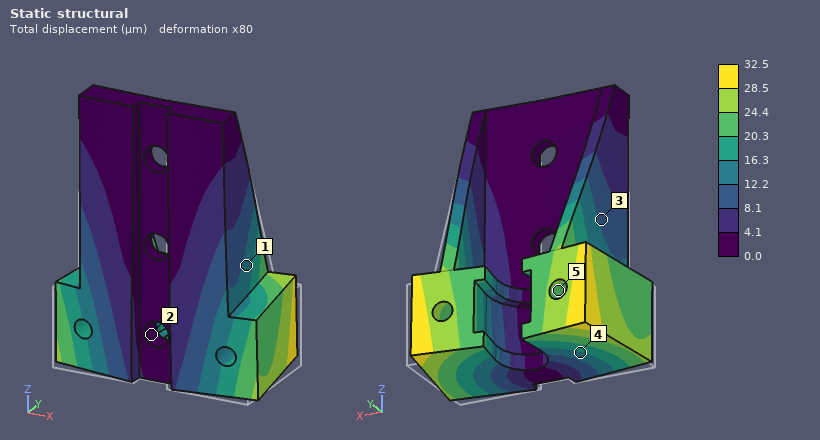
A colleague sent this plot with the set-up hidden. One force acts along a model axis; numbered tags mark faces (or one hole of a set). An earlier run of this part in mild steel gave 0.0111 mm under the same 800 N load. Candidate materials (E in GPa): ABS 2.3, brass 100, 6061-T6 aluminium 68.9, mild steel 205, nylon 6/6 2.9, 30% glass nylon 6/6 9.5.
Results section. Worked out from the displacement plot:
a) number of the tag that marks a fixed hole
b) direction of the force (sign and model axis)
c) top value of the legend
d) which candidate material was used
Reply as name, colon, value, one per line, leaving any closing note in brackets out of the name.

number of the tag that marks a fixed hole: 2
direction of the force: +Y
top value of the legend: 32.5 µm
which candidate material was used: 6061-T6 aluminium
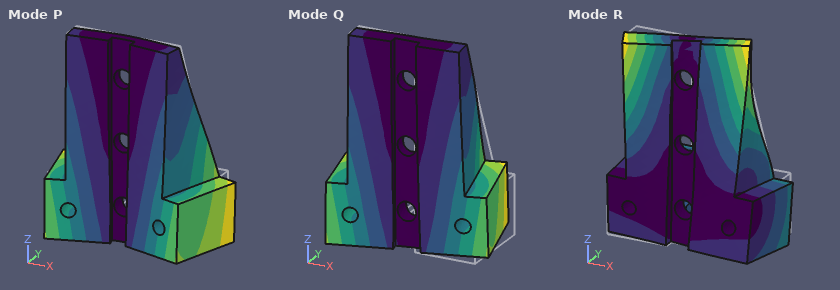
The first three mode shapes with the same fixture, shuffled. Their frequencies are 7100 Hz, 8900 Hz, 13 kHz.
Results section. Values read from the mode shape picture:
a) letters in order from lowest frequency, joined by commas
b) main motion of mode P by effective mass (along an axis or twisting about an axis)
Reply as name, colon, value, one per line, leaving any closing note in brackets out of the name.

letters in order from lowest frequency, joined by commas: Q, P, R
main motion of mode P by effective mass: along Y
